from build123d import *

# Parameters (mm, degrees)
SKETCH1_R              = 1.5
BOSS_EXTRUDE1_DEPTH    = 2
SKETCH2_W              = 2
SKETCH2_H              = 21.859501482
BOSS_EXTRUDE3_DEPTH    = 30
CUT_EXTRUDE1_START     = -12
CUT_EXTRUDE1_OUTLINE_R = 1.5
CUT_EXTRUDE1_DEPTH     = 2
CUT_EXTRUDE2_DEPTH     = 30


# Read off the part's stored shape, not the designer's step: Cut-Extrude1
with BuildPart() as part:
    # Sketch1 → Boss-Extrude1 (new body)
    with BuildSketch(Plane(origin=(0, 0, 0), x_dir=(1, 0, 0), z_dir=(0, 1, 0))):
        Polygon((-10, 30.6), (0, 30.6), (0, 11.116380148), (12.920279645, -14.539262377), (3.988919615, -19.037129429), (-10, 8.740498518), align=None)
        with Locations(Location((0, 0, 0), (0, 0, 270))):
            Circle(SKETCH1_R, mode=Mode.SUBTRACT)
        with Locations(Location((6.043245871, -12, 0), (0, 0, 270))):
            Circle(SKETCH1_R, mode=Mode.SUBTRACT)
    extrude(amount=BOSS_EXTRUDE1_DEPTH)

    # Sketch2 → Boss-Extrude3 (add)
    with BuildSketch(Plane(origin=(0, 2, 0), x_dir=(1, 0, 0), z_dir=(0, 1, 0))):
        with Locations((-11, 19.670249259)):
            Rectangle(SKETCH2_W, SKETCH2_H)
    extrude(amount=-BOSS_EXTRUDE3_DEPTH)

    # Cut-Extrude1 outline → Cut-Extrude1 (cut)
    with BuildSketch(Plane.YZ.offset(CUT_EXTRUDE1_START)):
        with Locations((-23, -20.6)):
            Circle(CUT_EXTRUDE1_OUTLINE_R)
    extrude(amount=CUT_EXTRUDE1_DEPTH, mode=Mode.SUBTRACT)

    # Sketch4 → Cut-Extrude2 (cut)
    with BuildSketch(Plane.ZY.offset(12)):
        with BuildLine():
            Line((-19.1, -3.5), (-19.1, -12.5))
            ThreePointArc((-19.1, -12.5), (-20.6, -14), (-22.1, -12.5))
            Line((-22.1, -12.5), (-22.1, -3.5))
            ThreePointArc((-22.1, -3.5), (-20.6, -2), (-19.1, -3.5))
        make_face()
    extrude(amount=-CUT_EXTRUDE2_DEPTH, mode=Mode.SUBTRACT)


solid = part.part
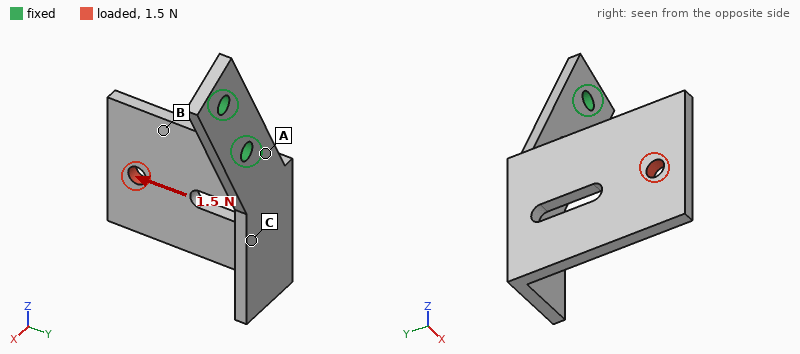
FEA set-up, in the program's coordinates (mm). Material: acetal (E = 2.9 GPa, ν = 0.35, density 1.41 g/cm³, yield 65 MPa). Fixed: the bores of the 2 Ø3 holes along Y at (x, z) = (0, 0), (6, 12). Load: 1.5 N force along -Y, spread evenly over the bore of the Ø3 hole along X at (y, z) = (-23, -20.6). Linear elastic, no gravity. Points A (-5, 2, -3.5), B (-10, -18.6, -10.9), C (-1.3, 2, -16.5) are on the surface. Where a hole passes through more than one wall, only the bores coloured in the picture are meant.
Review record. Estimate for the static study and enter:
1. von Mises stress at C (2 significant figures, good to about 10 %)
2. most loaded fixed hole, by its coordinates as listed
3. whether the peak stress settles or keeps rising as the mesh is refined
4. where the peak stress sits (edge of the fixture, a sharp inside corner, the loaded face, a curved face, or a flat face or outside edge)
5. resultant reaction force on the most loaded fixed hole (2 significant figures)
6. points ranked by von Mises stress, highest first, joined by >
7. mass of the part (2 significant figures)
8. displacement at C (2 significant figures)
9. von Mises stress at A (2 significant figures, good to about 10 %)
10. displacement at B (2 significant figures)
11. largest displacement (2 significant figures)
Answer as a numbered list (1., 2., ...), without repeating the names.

1. 0.94 MPa
2. (0, 0)
3. keeps rising
4. edge of the fixture
5. 1.6 N
6. A > C > B
7. 3.1 g
8. 0.14 mm
9. 3.9 MPa
10. 0.36 mm
11. 0.67 mm
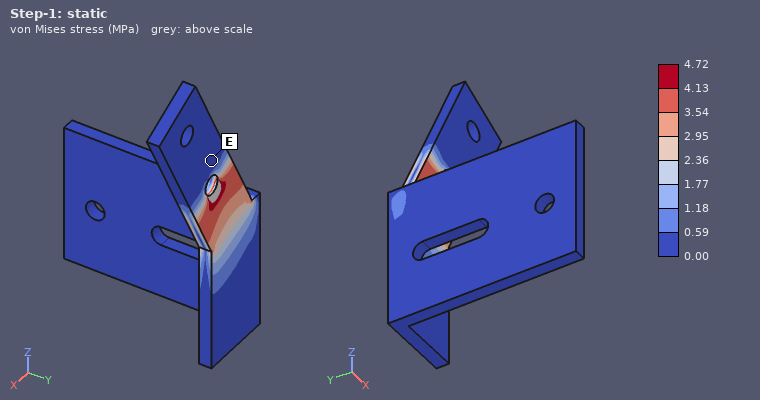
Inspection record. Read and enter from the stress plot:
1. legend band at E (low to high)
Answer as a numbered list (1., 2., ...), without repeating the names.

1. 0.00 to 0.59 MPa
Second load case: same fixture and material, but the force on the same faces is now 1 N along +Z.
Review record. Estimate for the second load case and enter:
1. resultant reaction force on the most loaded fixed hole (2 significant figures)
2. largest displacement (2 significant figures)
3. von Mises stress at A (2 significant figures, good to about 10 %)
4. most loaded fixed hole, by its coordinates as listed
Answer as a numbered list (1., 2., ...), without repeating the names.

1. 1.2 N
2. 0.64 mm
3. 3.3 MPa
4. (0, 0)
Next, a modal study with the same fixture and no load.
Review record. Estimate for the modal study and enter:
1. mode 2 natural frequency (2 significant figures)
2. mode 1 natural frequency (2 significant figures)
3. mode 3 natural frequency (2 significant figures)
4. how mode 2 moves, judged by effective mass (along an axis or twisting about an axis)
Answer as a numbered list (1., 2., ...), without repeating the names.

1. 260 Hz
2. 180 Hz
3. 920 Hz
4. along X
